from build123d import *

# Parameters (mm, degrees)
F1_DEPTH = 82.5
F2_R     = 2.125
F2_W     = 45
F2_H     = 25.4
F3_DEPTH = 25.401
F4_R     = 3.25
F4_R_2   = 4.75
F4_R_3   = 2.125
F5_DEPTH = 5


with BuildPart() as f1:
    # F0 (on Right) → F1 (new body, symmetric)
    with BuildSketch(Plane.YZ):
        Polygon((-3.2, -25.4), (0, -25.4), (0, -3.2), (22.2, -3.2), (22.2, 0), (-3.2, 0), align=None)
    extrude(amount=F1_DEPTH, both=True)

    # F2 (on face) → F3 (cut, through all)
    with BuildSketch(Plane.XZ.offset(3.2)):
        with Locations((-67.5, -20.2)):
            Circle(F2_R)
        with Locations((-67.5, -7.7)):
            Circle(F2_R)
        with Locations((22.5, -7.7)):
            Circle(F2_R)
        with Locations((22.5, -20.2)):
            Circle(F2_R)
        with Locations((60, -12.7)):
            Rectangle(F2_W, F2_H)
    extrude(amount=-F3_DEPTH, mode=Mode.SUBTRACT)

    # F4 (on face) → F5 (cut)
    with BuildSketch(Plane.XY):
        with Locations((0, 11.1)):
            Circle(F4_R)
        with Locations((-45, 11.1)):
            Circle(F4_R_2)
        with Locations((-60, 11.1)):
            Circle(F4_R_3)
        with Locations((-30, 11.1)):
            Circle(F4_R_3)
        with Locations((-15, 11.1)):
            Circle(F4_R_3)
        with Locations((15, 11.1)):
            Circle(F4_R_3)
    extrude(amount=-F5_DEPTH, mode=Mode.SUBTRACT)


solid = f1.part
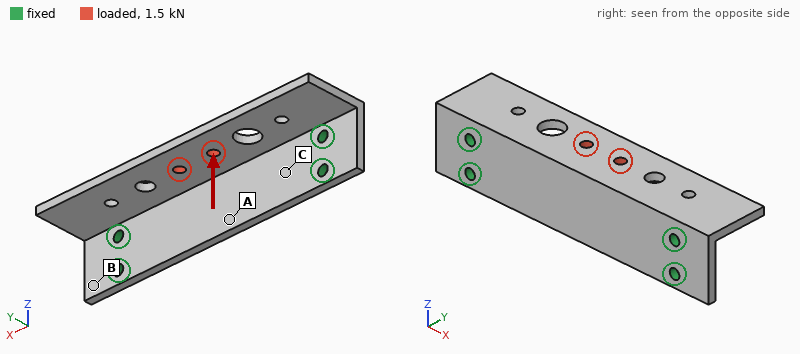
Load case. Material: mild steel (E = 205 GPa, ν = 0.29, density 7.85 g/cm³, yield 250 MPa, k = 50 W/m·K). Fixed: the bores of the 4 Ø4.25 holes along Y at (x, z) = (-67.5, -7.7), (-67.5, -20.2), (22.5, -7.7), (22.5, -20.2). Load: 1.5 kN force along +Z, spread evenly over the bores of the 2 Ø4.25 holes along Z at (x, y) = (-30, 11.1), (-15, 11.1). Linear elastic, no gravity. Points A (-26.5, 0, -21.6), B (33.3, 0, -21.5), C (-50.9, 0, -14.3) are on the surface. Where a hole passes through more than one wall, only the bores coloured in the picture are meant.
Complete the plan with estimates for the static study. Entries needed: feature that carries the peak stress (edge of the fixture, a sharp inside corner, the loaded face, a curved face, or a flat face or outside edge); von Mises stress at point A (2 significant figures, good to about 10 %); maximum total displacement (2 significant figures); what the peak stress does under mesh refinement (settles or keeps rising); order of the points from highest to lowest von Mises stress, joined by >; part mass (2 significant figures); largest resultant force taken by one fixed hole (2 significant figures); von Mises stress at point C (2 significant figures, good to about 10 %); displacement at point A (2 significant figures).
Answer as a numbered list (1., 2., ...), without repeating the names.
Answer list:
1. edge of the fixture
2. 41 MPa
3. 0.23 mm
4. keeps rising
5. C > A > B
6. 140 g
7. 1.2 kN
8. 100 MPa
9. 0.097 mm
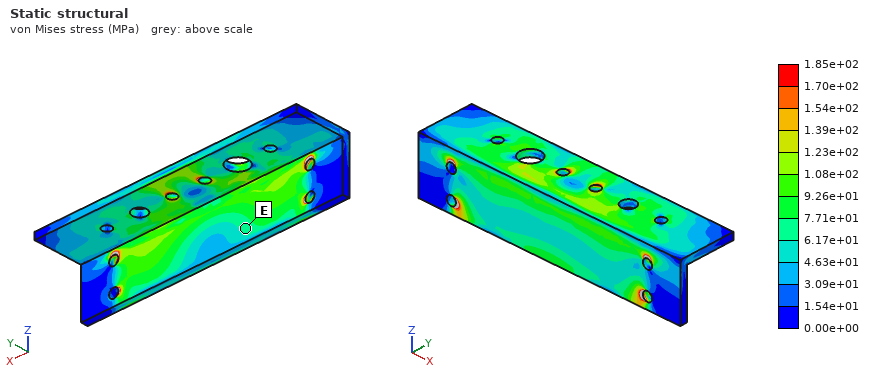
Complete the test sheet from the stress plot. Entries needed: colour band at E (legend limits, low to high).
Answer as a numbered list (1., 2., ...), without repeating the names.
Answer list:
1. 6.17e+01 to 7.71e+01 MPa
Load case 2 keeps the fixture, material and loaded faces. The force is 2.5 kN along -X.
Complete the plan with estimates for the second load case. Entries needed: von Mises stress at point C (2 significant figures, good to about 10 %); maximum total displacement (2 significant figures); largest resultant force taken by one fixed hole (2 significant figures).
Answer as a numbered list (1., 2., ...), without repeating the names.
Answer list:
1. 10 MPa
2. 9.9 µm
3. 980 N
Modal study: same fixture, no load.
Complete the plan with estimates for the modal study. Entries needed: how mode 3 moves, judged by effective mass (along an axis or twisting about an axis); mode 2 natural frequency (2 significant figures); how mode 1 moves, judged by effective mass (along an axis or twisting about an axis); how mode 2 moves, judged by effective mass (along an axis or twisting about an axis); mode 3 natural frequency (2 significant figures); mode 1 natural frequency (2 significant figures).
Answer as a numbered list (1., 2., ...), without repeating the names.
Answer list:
1. along Y
2. 3800 Hz
3. along Z
4. twisting about Y
5. 4200 Hz
6. 2500 Hz
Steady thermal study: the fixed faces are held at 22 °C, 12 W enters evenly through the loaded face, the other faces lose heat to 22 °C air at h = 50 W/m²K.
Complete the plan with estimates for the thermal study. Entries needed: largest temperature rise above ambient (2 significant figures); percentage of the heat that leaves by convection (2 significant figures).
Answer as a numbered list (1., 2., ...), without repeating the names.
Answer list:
1. 38 K
2. 53 %
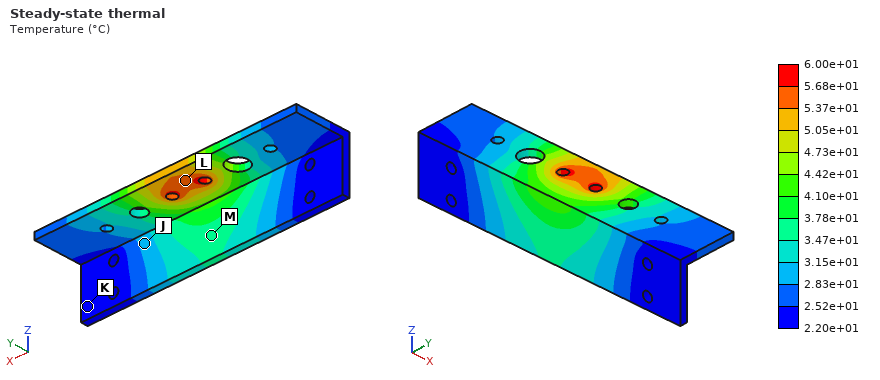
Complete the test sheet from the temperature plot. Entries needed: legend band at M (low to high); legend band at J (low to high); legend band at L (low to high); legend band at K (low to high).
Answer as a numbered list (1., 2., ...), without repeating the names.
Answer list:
1. 3.47e+01 to 3.78e+01 °C
2. 2.83e+01 to 3.15e+01 °C
3. 5.37e+01 to 5.68e+01 °C
4. 2.20e+01 to 2.52e+01 °C
